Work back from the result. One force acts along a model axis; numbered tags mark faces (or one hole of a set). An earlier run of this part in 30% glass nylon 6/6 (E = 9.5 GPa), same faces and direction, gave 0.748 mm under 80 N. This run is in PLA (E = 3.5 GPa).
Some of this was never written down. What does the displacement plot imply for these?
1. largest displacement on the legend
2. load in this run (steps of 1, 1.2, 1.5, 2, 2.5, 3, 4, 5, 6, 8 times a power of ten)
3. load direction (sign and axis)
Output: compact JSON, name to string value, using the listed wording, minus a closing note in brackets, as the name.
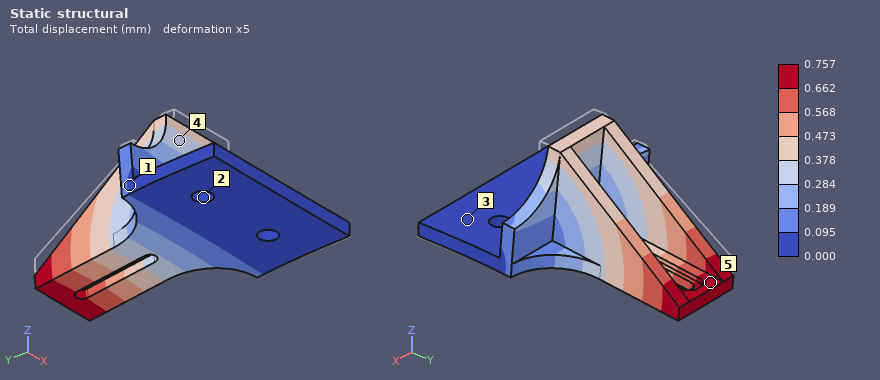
{"largest displacement on the legend": "0.757 mm", "load in this run": "30 N", "load direction": "-Z"}
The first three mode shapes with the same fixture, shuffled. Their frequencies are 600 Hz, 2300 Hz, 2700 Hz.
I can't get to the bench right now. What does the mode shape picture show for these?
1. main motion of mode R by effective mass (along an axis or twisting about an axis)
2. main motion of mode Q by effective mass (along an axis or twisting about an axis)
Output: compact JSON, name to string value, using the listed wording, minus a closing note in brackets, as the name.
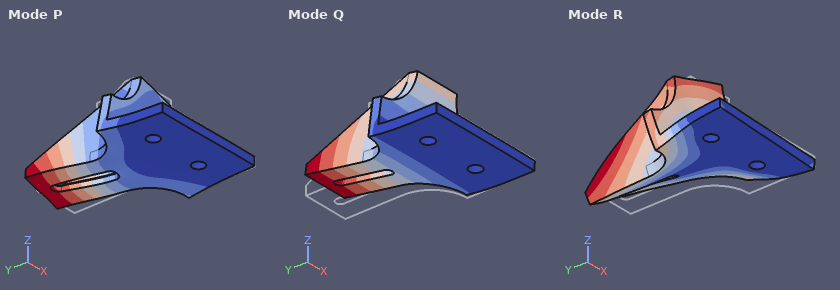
{"main motion of mode R by effective mass": "along X", "main motion of mode Q by effective mass": "along Z"}
